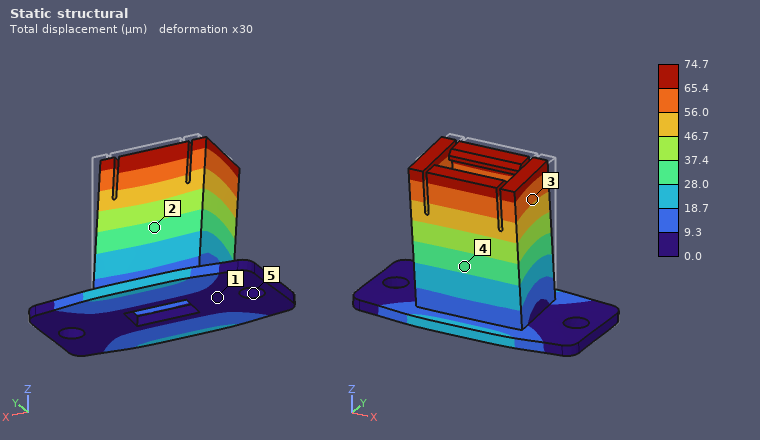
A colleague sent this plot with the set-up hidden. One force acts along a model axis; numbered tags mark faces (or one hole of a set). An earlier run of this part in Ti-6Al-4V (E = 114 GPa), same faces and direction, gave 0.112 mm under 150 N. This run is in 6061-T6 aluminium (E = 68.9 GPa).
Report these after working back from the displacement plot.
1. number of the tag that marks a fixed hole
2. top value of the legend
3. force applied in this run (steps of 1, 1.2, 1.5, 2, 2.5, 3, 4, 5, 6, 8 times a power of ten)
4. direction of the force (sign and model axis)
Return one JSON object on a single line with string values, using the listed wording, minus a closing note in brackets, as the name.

{"number of the tag that marks a fixed hole": "5", "top value of the legend": "74.7 µm", "force applied in this run": "60 N", "direction of the force": "-Y"}
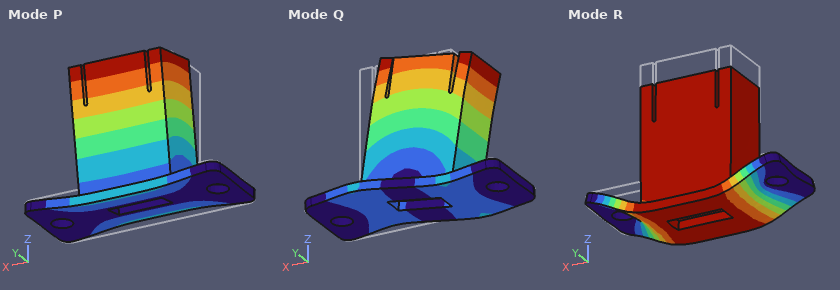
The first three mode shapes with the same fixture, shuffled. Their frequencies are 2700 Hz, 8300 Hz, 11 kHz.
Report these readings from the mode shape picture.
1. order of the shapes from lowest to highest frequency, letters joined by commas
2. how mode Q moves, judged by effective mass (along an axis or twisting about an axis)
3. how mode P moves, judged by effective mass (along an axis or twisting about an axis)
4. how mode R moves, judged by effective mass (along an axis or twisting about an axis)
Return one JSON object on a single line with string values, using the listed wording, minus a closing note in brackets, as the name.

{"order of the shapes from lowest to highest frequency, letters joined by commas": "P, Q, R", "how mode Q moves, judged by effective mass": "along X", "how mode P moves, judged by effective mass": "along Y", "how mode R moves, judged by effective mass": "along Z"}
